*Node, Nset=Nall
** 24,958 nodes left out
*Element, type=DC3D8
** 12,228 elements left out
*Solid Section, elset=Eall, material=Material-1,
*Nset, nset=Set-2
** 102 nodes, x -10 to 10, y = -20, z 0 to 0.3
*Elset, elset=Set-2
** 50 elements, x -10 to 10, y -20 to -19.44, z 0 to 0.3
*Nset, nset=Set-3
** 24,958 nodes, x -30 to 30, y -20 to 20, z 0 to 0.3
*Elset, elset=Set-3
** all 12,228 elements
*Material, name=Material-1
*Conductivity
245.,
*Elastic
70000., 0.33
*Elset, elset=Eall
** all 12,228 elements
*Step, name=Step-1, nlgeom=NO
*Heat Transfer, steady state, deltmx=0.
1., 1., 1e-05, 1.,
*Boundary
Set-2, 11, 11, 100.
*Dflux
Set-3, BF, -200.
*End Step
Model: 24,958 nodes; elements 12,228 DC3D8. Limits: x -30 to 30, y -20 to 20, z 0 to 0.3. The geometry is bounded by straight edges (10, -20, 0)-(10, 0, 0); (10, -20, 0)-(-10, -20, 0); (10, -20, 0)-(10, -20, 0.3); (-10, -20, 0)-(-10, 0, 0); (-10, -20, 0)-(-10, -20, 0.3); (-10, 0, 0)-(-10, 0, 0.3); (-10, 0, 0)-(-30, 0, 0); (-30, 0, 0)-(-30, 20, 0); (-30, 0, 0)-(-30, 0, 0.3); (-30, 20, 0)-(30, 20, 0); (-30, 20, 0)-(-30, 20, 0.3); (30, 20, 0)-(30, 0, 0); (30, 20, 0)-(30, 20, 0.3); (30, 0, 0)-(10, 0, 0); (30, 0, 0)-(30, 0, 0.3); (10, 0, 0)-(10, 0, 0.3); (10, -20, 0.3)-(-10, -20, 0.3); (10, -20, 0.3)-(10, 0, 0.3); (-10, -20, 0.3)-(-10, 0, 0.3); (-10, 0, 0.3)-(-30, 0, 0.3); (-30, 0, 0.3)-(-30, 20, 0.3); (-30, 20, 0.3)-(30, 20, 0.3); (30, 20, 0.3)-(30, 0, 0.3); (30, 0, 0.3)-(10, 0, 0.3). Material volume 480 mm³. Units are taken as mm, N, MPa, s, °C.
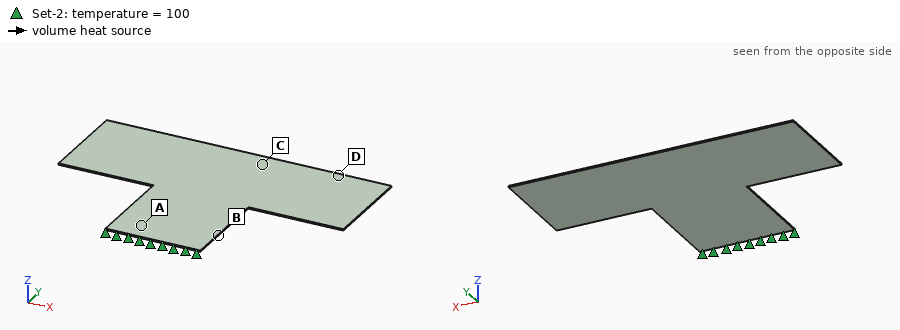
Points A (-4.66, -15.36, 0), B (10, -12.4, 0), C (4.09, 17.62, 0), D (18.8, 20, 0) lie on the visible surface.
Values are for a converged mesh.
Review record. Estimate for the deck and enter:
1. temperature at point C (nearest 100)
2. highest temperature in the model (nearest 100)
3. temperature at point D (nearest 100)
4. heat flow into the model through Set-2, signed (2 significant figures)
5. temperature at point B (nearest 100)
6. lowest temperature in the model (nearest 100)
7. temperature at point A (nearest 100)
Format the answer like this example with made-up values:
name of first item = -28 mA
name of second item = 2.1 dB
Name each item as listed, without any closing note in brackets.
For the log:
temperature at point C = -1400 °C
highest temperature in the model = 100 °C
temperature at point D = -1500 °C
heat flow into the model through Set-2, signed = 96000 mW
temperature at point B = -400 °C
lowest temperature in the model = -1500 °C
temperature at point A = -200 °C
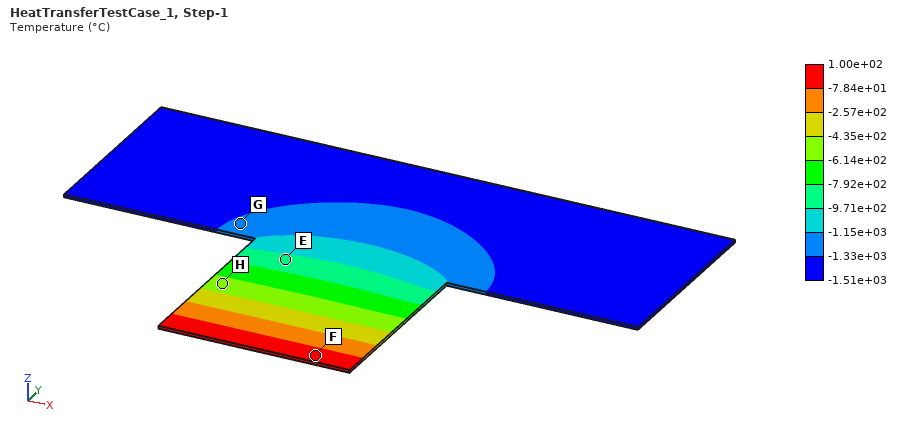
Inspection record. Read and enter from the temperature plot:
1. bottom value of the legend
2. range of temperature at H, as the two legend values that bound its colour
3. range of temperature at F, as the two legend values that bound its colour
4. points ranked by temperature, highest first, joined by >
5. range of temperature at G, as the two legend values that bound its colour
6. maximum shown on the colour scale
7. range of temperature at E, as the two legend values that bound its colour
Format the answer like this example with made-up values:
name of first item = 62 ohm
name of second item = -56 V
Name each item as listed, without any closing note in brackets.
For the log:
bottom value of the legend = -1.51e+03 °C
range of temperature at H, as the two legend values that bound its colour = -6.14e+02 to -4.35e+02 °C
range of temperature at F, as the two legend values that bound its colour = -7.84e+01 to 1.00e+02 °C
points ranked by temperature, highest first, joined by > = F > H > E > G
range of temperature at G, as the two legend values that bound its colour = -1.33e+03 to -1.15e+03 °C
maximum shown on the colour scale = 1.00e+02 °C
range of temperature at E, as the two legend values that bound its colour = -9.71e+02 to -7.92e+02 °C
